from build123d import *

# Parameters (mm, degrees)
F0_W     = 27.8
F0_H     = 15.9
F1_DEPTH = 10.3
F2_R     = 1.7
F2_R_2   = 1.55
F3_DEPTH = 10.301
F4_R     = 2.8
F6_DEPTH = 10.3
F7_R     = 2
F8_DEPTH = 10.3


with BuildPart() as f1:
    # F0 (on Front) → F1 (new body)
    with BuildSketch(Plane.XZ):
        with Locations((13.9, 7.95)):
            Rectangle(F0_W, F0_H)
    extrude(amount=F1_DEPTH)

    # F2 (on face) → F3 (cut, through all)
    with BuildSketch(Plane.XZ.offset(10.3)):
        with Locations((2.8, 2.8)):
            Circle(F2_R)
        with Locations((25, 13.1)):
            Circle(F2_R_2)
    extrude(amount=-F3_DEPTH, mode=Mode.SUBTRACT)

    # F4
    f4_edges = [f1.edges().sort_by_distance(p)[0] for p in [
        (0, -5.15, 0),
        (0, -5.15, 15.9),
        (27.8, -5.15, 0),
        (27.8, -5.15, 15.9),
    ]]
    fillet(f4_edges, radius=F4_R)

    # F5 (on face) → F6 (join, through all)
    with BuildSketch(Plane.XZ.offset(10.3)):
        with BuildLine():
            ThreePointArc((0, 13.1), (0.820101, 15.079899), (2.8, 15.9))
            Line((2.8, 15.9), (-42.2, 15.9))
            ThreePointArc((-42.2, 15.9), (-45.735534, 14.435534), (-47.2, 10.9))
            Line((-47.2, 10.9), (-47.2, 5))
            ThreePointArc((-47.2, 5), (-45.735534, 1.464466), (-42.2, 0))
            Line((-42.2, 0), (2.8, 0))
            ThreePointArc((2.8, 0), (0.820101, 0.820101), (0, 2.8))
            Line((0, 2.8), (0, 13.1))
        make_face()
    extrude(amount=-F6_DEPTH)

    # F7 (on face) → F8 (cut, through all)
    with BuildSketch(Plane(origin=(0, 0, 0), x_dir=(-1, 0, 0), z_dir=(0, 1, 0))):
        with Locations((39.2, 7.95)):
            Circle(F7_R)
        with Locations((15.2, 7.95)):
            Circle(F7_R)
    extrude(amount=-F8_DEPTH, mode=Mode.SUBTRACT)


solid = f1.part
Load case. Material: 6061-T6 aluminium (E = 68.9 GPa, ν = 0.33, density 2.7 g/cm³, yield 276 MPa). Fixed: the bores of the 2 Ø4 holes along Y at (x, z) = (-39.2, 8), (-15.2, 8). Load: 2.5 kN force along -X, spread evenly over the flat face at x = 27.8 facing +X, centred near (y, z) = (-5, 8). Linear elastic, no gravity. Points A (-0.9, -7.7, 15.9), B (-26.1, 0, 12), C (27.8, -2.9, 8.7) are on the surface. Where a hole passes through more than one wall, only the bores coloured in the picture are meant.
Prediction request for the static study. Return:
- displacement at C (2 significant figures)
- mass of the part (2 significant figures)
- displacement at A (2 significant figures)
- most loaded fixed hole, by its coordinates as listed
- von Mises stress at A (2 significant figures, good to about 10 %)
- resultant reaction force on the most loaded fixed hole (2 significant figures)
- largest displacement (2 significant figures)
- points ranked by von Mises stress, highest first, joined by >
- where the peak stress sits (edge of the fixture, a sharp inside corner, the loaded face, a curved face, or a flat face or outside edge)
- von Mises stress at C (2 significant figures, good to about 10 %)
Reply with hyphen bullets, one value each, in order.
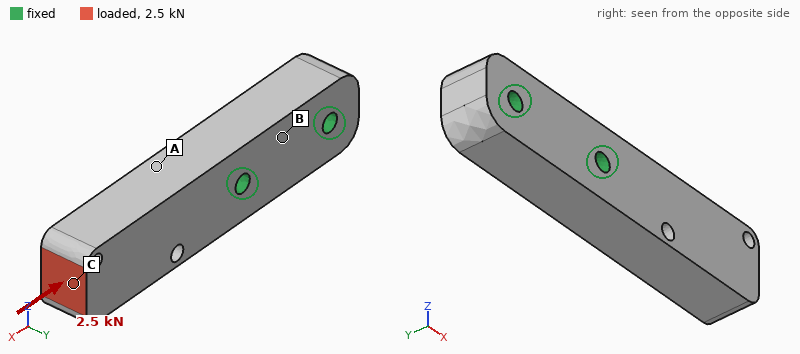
- 12 µm
- 32 g
- 3.5 µm
- (-15.2, 8)
- 13 MPa
- 2.3 kN
- 12 µm
- C > A > B
- a curved face
- 24 MPa
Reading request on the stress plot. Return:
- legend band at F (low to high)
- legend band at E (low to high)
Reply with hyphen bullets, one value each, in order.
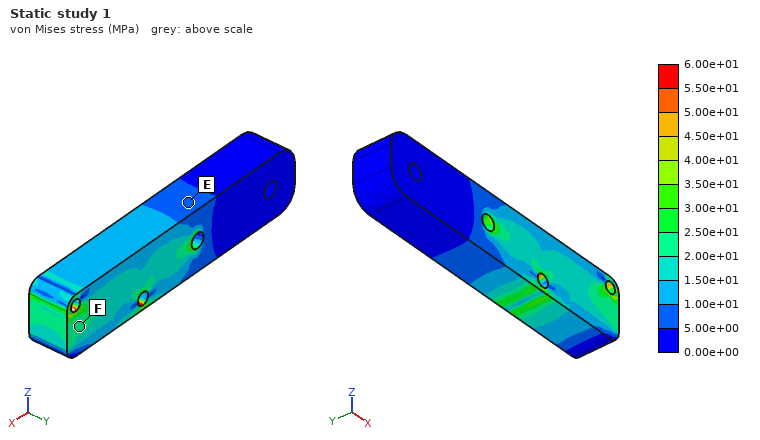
- 2.00e+01 to 2.50e+01 MPa
- 5.00e+00 to 1.00e+01 MPa
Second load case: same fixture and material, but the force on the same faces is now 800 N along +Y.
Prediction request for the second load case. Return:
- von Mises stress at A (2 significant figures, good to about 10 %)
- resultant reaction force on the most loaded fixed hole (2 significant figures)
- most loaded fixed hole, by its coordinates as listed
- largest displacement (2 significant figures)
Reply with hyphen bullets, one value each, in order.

- 44 MPa
- 1.1 kN
- (-15.2, 8)
- 0.24 mm
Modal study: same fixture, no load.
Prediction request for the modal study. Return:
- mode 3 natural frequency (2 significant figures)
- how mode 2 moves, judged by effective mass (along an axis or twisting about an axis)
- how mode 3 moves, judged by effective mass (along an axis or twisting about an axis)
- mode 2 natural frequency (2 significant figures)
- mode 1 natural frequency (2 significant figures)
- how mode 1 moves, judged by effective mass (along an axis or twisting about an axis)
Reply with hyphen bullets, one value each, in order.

- 15 kHz
- along Z
- twisting about X
- 5300 Hz
- 4300 Hz
- along Y
